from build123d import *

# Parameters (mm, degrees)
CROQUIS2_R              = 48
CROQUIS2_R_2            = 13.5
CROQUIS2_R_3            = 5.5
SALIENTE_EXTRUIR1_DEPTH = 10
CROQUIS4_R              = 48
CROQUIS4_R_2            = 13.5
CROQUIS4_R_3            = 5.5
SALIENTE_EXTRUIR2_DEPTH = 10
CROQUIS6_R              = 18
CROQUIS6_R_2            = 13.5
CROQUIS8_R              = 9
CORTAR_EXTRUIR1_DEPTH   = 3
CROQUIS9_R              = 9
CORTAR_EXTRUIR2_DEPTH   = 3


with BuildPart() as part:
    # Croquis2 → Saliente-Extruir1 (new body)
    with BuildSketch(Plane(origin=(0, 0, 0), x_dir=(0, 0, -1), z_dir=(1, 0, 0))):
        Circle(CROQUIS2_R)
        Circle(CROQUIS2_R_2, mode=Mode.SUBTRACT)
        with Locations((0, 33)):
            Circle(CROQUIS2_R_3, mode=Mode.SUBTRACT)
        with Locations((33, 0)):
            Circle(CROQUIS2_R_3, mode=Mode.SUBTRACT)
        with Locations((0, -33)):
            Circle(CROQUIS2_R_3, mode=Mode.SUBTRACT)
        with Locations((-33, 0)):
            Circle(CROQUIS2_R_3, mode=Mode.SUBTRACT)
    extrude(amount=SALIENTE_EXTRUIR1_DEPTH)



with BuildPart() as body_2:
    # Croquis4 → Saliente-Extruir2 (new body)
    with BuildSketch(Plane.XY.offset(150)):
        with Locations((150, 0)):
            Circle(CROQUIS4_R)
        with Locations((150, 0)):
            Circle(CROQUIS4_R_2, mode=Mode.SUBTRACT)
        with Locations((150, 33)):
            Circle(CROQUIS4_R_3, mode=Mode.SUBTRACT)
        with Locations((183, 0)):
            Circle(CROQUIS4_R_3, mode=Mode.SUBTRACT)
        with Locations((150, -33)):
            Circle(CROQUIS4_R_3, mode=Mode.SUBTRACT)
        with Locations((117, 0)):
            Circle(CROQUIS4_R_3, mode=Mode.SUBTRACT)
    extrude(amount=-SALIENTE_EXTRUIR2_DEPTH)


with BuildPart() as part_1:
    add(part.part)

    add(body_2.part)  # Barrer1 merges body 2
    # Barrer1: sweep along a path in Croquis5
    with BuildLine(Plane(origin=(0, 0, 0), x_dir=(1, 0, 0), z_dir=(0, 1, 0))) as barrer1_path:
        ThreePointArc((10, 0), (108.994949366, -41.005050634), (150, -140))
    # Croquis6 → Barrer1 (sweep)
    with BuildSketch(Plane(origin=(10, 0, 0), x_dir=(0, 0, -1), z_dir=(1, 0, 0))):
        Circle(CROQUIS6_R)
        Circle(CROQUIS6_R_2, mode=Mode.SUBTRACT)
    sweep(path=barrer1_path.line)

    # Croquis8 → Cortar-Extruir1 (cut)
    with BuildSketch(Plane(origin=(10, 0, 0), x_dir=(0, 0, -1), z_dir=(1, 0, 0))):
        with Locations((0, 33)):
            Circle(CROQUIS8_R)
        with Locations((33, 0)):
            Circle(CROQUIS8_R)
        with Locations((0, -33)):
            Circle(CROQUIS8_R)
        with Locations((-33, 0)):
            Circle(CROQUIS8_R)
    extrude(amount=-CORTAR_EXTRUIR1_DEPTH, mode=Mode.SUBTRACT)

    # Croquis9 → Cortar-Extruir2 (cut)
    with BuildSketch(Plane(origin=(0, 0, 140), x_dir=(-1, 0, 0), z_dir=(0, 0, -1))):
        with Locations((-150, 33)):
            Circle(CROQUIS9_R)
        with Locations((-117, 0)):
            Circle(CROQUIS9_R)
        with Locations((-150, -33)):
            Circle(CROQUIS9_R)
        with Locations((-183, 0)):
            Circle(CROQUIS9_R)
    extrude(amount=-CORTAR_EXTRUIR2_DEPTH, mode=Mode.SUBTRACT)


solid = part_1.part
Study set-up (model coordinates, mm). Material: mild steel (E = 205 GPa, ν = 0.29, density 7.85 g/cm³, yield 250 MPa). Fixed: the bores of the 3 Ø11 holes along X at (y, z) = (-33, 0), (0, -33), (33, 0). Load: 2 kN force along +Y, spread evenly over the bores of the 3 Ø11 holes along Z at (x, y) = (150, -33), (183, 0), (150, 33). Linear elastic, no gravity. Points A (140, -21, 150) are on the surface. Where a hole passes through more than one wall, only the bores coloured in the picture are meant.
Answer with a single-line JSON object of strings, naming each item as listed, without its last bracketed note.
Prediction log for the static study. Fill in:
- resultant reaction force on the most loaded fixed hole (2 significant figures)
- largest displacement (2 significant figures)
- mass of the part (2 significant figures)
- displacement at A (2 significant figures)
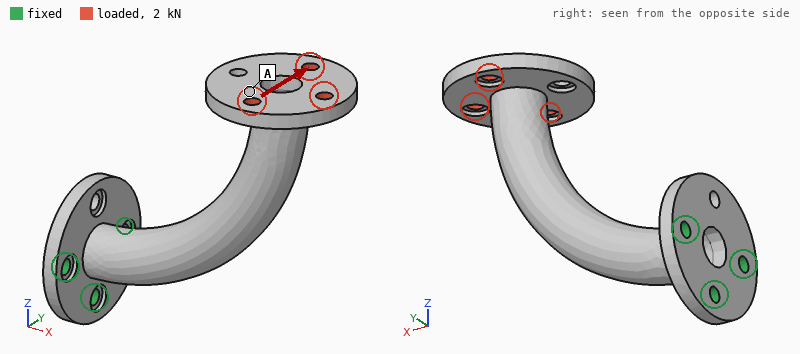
{"resultant reaction force on the most loaded fixed hole": "7.0 kN", "largest displacement": "1.00 mm", "mass of the part": "1.7 kg", "displacement at A": "0.82 mm"}
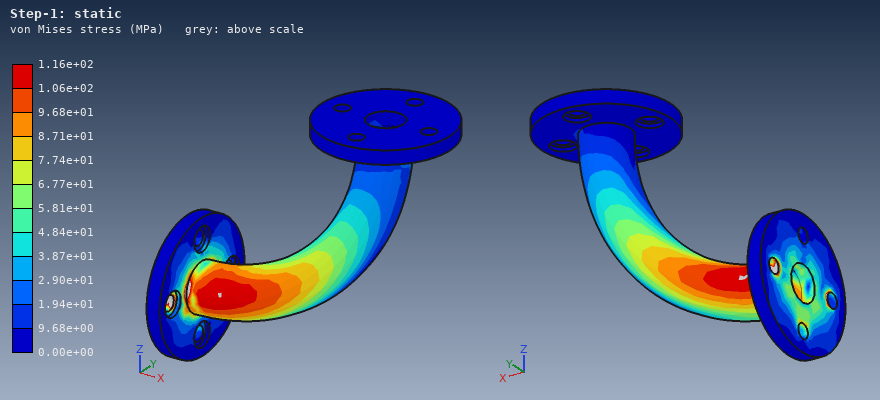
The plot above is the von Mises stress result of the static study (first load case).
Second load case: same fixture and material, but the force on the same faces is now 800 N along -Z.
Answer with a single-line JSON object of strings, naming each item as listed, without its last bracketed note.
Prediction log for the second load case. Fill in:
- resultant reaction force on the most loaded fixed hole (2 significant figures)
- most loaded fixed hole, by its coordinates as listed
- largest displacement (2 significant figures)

{"resultant reaction force on the most loaded fixed hole": "3.4 kN", "most loaded fixed hole, by its coordinates as listed": "(0, -33)", "largest displacement": "0.34 mm"}
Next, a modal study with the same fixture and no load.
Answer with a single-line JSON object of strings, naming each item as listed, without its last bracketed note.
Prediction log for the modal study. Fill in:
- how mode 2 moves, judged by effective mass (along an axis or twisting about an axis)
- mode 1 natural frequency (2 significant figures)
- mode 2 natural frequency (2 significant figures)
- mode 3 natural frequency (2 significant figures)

{"how mode 2 moves, judged by effective mass": "along Y", "mode 1 natural frequency": "260 Hz", "mode 2 natural frequency": "310 Hz", "mode 3 natural frequency": "1200 Hz"}
